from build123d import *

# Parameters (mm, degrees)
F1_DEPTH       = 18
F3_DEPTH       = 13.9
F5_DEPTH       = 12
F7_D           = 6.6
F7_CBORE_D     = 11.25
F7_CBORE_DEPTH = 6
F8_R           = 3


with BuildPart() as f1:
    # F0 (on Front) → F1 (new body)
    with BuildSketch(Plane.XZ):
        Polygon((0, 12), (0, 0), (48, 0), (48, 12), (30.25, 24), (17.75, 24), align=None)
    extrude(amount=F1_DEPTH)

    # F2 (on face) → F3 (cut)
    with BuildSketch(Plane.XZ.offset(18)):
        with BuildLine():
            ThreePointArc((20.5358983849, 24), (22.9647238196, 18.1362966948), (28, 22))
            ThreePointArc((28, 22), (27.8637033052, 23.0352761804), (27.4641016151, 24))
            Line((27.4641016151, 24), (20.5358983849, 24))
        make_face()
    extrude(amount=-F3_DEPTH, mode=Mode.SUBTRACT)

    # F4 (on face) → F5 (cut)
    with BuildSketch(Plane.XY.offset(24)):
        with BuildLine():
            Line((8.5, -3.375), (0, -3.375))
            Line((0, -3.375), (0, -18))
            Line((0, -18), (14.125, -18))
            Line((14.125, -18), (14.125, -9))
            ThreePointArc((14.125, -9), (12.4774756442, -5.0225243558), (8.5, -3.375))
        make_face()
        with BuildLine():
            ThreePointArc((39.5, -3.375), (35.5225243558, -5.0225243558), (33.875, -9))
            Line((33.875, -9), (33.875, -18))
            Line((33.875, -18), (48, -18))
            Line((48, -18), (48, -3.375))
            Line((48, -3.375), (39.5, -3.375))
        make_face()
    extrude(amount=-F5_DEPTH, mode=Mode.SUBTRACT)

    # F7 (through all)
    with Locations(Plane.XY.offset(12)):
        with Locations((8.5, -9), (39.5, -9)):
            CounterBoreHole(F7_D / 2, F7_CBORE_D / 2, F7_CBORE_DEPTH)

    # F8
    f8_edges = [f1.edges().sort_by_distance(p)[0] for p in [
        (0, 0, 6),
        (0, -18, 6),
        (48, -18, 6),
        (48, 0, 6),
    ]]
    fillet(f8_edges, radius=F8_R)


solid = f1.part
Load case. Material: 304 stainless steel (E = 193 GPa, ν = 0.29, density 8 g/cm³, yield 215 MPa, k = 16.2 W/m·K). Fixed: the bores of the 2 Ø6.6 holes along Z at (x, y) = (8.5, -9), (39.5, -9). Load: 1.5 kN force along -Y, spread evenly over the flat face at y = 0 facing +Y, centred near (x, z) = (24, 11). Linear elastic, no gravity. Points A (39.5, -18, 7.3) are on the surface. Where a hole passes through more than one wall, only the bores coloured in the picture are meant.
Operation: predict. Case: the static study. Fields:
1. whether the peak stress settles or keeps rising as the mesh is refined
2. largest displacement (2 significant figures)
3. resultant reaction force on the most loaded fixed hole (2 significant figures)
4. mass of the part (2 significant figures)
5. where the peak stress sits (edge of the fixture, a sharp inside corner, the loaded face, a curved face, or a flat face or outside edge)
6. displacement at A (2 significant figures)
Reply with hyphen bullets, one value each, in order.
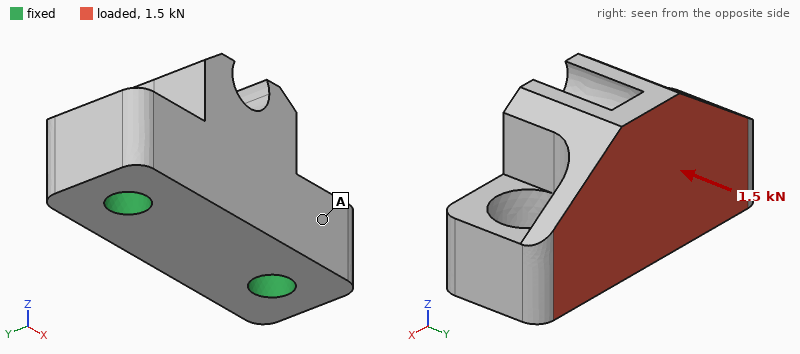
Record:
- keeps rising
- 4.9 µm
- 750 N
- 100 g
- edge of the fixture
- 1.2 µm
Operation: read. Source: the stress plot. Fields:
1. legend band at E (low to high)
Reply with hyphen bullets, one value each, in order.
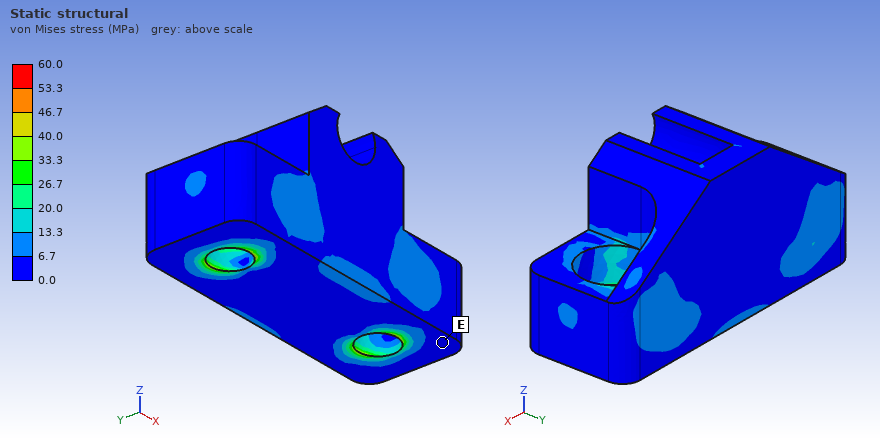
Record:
- 0.0 to 6.7 MPa
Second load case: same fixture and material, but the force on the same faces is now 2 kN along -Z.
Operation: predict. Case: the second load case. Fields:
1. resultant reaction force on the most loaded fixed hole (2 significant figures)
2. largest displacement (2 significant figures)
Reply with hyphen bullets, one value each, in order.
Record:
- 1.0 kN
- 6.4 µm
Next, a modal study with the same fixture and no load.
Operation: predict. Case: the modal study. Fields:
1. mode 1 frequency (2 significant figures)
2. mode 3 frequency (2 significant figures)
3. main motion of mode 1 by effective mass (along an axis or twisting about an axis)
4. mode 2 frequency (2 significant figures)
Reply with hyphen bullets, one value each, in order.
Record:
- 12 kHz
- 27 kHz
- along Y
- 26 kHz
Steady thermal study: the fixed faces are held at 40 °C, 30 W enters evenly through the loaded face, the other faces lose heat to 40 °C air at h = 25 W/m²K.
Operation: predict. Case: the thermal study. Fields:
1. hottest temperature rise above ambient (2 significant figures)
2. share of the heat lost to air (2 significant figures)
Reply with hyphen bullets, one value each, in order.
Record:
- 67 K
- 8.9 %
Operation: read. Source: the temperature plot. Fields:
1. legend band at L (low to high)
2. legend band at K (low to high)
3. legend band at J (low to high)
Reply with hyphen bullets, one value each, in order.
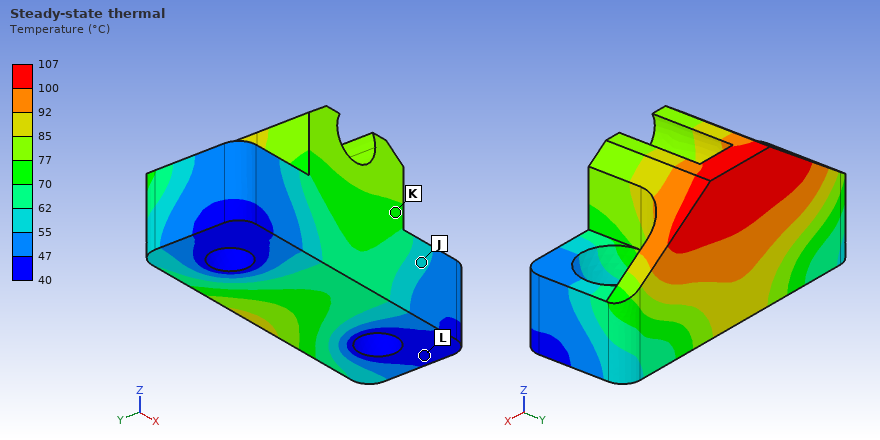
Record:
- 40 to 47 °C
- 70 to 77 °C
- 55 to 62 °C
